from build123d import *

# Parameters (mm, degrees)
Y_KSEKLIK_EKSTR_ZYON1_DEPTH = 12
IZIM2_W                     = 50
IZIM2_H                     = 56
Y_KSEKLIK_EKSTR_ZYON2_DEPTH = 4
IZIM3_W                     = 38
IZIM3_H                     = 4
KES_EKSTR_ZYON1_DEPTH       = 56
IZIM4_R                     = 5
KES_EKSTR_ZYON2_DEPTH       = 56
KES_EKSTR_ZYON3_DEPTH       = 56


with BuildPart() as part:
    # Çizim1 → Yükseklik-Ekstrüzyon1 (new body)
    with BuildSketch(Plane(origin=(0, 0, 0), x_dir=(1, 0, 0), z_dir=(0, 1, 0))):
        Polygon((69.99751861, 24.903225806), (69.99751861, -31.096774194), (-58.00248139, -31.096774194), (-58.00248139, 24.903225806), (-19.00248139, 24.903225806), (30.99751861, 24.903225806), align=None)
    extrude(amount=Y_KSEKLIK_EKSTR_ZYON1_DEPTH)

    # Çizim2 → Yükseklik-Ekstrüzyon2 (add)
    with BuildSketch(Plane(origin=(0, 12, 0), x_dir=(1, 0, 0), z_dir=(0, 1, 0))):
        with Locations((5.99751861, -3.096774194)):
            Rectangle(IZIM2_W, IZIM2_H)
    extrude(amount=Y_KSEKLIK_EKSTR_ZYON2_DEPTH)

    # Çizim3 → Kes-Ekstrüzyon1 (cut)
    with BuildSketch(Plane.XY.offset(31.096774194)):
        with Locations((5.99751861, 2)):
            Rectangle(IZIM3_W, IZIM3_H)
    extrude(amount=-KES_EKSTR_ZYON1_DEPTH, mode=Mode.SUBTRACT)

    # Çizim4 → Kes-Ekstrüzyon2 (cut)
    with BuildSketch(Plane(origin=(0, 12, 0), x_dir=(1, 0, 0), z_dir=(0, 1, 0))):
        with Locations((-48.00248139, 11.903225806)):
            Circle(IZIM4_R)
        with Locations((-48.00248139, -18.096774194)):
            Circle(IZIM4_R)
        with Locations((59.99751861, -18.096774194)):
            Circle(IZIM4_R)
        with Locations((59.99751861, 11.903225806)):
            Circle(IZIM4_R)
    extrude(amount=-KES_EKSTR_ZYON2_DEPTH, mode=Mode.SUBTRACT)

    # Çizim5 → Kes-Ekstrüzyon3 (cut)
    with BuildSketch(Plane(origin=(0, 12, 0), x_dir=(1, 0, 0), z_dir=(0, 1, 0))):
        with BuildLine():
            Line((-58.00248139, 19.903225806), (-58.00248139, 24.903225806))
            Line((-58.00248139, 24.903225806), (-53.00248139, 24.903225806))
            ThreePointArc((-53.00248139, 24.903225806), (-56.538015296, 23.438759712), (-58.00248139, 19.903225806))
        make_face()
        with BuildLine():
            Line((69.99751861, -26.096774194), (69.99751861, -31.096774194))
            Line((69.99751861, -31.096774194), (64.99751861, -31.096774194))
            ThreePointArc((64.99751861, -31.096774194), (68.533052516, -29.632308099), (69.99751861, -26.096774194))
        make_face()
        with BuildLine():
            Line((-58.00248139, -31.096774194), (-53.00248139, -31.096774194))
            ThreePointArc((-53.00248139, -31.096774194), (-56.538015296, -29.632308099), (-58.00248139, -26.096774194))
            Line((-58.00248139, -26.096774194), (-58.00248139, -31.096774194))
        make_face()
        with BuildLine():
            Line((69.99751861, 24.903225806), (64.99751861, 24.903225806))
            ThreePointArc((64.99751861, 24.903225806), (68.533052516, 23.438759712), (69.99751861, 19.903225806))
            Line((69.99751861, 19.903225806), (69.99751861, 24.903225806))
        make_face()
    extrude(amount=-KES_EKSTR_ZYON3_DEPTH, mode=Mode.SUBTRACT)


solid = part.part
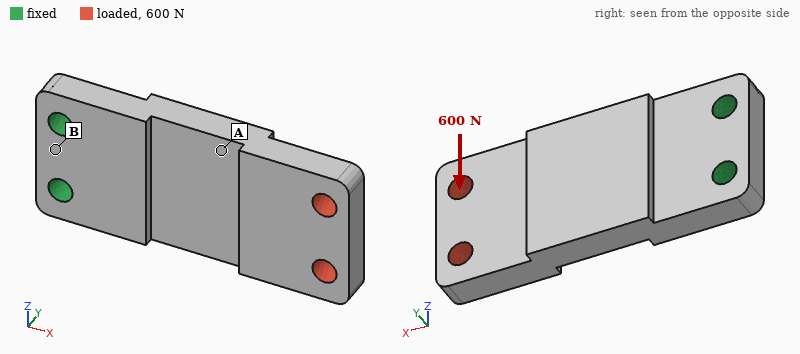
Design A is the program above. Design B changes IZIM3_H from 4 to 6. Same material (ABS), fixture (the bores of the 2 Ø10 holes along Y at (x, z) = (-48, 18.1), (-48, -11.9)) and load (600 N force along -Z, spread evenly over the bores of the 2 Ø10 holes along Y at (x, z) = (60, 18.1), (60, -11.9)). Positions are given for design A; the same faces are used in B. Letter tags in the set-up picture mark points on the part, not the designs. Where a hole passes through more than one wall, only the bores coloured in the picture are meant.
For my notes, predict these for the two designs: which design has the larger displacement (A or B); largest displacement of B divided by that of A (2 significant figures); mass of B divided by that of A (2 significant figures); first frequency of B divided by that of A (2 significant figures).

B
1.1
0.97
0.96
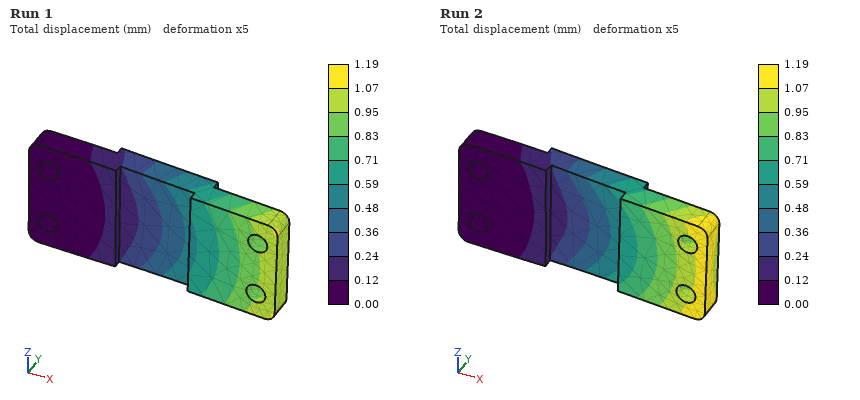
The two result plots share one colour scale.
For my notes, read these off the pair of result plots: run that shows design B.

Run 2
